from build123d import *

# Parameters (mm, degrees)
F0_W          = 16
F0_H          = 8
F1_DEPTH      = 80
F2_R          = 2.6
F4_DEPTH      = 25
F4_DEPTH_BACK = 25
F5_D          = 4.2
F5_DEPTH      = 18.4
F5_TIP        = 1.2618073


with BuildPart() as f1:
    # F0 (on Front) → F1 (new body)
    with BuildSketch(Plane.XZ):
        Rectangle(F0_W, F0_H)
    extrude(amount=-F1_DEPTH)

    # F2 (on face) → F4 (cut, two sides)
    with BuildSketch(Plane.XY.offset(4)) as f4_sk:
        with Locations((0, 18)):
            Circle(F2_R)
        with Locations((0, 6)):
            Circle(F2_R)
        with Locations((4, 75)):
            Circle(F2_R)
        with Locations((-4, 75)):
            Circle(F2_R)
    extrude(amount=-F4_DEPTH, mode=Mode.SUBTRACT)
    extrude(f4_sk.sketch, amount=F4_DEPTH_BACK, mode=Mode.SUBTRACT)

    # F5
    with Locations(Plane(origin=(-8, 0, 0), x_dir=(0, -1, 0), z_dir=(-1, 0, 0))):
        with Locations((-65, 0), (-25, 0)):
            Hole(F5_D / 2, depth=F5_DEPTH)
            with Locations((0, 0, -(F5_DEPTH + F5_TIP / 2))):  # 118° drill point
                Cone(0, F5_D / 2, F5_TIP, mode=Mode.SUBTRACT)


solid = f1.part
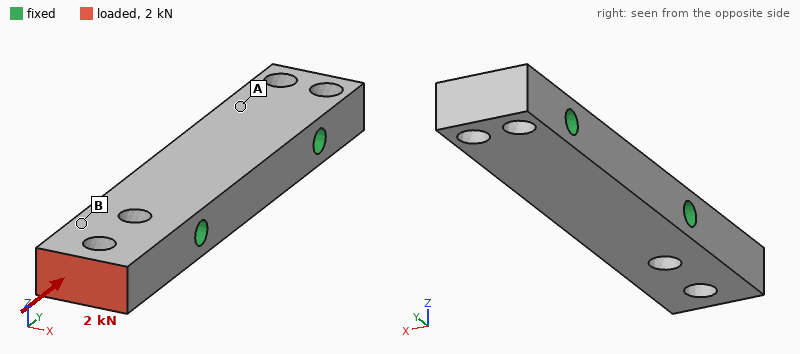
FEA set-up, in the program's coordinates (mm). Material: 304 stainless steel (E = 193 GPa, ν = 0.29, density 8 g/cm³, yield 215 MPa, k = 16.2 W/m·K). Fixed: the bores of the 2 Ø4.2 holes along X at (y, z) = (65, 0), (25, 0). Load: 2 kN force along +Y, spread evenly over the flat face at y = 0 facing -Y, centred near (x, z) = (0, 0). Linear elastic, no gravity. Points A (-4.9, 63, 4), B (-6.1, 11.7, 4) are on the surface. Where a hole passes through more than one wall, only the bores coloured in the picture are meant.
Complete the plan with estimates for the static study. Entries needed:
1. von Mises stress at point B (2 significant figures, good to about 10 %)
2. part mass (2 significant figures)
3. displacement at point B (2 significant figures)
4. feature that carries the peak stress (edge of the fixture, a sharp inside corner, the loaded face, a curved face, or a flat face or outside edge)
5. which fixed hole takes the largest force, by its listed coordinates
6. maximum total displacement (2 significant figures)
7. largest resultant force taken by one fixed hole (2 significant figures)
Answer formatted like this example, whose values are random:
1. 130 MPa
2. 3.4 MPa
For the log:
1. 22 MPa
2. 73 g
3. 1.3 µm
4. a curved face
5. (25, 0)
6. 3.0 µm
7. 2.0 kN
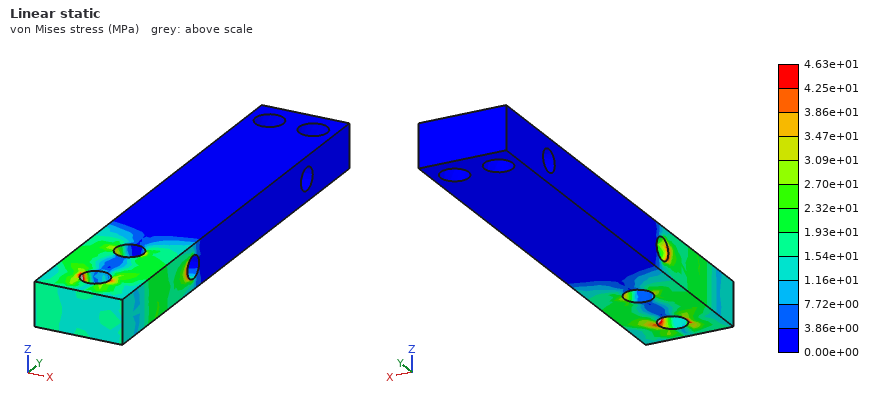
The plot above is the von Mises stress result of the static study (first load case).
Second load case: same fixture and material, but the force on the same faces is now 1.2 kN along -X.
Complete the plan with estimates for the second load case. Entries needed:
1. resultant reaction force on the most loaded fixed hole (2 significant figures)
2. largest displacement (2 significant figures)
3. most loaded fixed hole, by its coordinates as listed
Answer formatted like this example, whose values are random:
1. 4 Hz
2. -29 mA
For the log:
1. 1.2 kN
2. 18 µm
3. (25, 0)
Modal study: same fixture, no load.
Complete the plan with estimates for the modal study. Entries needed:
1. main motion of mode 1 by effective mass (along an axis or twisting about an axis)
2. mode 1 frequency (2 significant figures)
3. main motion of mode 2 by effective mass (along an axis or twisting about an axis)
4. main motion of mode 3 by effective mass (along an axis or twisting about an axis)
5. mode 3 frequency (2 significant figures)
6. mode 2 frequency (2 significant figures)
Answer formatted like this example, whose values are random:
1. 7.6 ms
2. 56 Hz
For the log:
1. along Z
2. 9000 Hz
3. along X
4. along Z
5. 21 kHz
6. 16 kHz
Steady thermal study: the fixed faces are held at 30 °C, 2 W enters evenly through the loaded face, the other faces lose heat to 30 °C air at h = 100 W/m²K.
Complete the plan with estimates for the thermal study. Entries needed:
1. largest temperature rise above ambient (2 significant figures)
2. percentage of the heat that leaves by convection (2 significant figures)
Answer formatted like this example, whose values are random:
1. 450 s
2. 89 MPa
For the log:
1. 19 K
2. 52 %
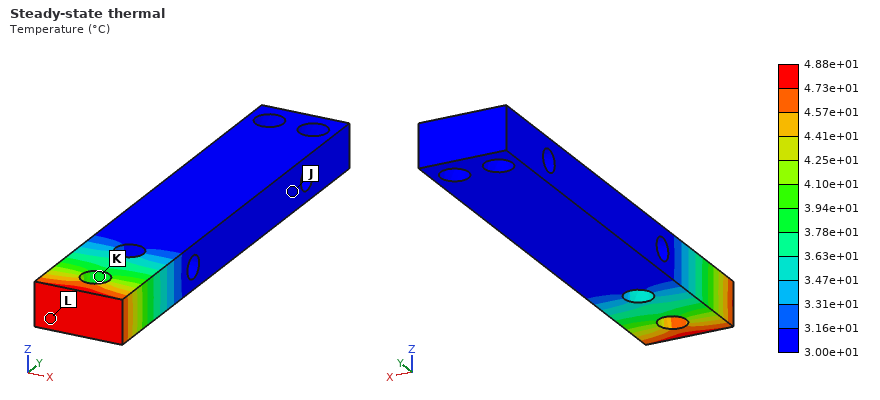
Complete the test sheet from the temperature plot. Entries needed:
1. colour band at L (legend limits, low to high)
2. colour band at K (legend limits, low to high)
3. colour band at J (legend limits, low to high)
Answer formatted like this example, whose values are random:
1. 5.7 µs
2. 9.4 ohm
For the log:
1. 4.73e+01 to 4.88e+01 °C
2. 3.78e+01 to 3.94e+01 °C
3. 3.00e+01 to 3.16e+01 °C
